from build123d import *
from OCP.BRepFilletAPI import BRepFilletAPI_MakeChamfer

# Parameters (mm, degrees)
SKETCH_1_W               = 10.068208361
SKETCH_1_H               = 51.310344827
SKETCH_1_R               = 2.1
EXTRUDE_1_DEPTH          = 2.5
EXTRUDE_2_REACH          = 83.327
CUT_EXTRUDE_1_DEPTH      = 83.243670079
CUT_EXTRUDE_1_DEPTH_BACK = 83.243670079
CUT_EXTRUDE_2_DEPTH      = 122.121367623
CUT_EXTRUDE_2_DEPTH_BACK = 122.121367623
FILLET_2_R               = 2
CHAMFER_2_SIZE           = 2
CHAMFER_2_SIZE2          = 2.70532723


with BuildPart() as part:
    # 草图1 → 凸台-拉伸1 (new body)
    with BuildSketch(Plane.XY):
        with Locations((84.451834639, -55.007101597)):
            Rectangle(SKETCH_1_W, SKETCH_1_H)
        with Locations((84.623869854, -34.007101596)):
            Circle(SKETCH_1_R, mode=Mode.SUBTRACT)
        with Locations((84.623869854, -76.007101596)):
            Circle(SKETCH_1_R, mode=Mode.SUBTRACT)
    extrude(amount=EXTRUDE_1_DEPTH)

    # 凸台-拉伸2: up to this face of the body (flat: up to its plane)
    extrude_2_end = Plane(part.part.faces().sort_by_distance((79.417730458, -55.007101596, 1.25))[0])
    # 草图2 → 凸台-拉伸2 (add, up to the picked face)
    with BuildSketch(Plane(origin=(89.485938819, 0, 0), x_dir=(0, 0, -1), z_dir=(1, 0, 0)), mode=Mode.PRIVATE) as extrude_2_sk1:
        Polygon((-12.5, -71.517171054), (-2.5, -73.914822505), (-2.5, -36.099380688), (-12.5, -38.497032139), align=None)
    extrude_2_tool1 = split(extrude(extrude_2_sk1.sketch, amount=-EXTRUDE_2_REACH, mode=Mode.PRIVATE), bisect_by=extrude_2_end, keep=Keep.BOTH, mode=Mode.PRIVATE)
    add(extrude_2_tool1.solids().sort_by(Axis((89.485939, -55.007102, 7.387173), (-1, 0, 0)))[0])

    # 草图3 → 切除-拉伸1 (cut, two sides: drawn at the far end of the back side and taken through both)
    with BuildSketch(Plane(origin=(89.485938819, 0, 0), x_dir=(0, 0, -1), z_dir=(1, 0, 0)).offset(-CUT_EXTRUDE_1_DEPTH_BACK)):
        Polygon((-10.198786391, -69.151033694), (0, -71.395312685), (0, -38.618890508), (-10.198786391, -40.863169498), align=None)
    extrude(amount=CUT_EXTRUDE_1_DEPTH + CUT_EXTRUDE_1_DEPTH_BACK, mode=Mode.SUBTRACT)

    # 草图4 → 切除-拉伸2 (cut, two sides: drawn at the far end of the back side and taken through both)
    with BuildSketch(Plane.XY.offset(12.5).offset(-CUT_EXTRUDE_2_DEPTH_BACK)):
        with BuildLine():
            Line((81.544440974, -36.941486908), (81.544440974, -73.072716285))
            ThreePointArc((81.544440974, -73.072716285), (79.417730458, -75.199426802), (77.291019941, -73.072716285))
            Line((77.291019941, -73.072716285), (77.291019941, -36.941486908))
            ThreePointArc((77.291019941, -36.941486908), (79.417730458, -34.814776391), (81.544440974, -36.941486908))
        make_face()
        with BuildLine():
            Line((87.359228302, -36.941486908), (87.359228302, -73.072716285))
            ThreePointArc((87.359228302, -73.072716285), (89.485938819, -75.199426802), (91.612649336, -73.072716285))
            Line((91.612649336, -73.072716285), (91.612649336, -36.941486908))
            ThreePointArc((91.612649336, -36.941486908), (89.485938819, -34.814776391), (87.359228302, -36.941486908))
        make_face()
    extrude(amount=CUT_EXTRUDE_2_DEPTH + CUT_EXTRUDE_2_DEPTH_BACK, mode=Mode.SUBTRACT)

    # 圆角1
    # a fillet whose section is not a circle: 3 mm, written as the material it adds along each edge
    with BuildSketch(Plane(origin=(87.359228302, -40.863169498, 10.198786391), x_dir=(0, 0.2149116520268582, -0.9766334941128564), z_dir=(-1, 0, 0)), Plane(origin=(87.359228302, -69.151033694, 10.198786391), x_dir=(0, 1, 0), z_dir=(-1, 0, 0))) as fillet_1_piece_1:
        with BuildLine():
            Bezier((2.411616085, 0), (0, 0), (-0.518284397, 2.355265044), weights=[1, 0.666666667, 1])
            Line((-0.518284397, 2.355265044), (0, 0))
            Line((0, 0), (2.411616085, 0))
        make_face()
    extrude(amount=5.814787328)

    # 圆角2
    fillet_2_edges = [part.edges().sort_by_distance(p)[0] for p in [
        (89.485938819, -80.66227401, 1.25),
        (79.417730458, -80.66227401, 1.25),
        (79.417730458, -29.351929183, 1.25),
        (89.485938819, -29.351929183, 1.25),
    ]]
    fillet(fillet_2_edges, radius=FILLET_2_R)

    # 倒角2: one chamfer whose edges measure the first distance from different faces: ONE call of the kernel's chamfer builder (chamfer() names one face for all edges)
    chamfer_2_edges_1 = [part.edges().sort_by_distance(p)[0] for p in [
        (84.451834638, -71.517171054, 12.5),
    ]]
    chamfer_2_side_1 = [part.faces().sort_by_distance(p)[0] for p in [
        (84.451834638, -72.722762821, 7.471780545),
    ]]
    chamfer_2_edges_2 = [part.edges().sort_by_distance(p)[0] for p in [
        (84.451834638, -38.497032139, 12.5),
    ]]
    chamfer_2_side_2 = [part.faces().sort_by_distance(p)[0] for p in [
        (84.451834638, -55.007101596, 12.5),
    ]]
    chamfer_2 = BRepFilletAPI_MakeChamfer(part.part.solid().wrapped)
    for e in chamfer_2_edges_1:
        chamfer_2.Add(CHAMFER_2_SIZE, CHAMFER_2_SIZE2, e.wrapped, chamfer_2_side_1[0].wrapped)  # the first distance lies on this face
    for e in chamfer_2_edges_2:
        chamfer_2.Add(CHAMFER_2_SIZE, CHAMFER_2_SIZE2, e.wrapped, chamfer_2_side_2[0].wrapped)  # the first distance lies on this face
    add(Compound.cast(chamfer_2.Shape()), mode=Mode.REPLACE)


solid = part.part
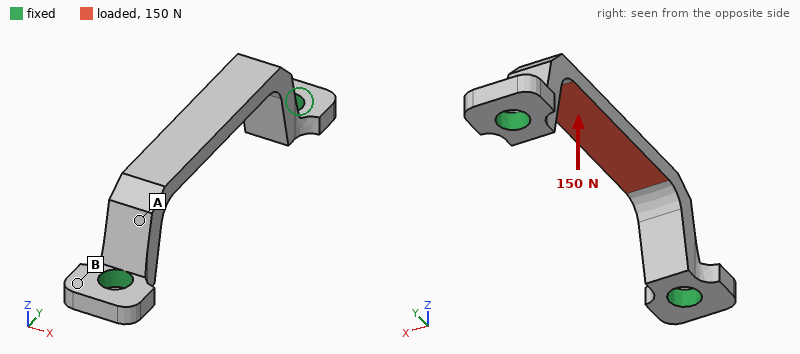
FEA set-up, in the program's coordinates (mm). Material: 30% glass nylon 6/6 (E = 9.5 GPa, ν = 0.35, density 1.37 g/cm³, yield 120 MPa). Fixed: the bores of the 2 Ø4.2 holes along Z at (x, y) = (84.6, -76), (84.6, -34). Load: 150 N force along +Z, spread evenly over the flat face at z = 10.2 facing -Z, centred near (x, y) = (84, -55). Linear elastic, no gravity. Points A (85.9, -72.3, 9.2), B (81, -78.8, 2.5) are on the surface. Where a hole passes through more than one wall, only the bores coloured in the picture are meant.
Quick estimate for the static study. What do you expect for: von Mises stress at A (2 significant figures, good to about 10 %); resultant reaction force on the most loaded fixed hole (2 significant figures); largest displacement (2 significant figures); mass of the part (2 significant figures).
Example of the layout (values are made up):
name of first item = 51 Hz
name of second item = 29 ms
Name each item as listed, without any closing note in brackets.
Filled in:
von Mises stress at A = 23 MPa
resultant reaction force on the most loaded fixed hole = 110 N
largest displacement = 0.27 mm
mass of the part = 1.4 g
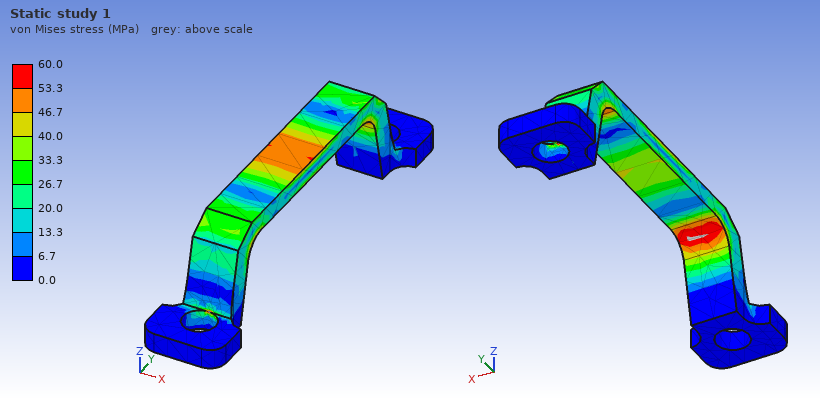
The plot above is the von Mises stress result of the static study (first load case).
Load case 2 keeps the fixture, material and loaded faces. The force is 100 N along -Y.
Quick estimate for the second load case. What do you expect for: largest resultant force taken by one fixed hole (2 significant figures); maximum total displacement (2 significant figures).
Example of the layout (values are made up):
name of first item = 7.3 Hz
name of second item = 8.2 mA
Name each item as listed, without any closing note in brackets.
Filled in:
largest resultant force taken by one fixed hole = 51 N
maximum total displacement = 0.13 mm
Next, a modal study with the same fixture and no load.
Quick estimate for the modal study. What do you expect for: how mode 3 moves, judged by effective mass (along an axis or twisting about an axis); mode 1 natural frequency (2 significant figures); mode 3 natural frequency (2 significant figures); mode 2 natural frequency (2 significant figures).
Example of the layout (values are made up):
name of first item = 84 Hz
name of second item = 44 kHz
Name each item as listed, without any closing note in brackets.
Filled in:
how mode 3 moves, judged by effective mass = along Z
mode 1 natural frequency = 5300 Hz
mode 3 natural frequency = 6400 Hz
mode 2 natural frequency = 5500 Hz
